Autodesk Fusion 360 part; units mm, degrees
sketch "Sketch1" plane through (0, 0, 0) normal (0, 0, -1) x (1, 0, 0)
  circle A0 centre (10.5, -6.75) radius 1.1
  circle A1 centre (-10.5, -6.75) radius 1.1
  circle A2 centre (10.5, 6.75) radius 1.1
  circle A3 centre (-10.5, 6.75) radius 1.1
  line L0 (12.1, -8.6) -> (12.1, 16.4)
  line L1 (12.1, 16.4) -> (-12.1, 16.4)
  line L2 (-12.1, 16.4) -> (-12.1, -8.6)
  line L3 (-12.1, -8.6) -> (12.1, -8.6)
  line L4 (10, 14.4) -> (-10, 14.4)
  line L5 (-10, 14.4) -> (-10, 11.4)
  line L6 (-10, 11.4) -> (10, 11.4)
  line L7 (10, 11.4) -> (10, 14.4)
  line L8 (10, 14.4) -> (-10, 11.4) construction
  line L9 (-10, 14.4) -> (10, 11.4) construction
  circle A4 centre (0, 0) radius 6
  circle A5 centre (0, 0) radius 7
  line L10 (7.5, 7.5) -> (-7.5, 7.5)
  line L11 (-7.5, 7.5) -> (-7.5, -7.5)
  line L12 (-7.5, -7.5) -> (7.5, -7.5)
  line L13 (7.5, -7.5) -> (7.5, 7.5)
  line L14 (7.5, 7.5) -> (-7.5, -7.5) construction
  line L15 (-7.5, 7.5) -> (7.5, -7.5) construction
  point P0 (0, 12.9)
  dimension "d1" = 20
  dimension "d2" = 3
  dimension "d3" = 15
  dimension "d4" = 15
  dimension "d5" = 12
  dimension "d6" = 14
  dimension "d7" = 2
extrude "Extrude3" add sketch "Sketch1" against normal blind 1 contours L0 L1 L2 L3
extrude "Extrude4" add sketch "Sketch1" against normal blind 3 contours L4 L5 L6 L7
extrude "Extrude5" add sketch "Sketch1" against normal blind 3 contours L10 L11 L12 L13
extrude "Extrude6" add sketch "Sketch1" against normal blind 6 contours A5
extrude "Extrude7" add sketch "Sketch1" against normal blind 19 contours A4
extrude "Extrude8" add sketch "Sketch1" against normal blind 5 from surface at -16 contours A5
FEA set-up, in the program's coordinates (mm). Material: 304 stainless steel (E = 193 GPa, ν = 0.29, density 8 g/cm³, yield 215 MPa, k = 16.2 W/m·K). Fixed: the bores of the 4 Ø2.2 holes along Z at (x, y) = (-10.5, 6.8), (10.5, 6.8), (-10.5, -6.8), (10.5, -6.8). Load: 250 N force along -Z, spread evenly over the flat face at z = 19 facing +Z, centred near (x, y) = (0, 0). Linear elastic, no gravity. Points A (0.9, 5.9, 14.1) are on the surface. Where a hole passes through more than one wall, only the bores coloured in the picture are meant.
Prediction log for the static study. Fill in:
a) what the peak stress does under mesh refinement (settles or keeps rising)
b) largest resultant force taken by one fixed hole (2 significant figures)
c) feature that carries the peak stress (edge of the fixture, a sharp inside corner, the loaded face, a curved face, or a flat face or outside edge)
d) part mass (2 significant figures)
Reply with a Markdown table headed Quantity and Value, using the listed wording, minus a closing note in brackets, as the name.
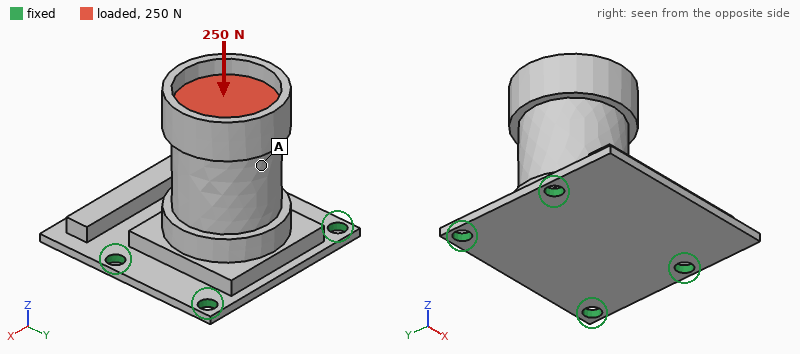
| Quantity | Value |
|---|---|
| what the peak stress does under mesh refinement | keeps rising |
| largest resultant force taken by one fixed hole | 82 N |
| feature that carries the peak stress | edge of the fixture |
| part mass | 26 g |
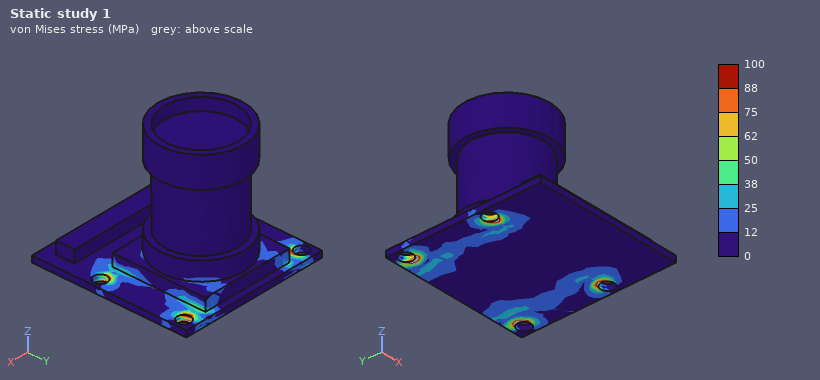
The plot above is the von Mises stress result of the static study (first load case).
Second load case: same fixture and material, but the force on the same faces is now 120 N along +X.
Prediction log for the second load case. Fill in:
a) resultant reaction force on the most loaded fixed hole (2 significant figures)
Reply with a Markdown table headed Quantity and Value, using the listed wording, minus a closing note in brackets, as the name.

| Quantity | Value |
|---|---|
| resultant reaction force on the most loaded fixed hole | 75 N |
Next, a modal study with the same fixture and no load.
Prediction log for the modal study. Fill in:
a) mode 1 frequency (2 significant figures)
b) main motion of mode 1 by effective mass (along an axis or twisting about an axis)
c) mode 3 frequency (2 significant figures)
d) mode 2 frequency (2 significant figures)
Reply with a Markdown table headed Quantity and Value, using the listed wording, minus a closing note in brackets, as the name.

| Quantity | Value |
|---|---|
| mode 1 frequency | 5700 Hz |
| main motion of mode 1 by effective mass | along Y |
| mode 3 frequency | 7800 Hz |
| mode 2 frequency | 7800 Hz |
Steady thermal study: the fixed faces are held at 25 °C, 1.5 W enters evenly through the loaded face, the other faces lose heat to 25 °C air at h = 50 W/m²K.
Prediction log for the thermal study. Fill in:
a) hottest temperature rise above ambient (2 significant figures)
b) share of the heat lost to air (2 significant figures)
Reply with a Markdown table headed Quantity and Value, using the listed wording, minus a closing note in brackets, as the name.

| Quantity | Value |
|---|---|
| hottest temperature rise above ambient | 17 K |
| share of the heat lost to air | 55 % |
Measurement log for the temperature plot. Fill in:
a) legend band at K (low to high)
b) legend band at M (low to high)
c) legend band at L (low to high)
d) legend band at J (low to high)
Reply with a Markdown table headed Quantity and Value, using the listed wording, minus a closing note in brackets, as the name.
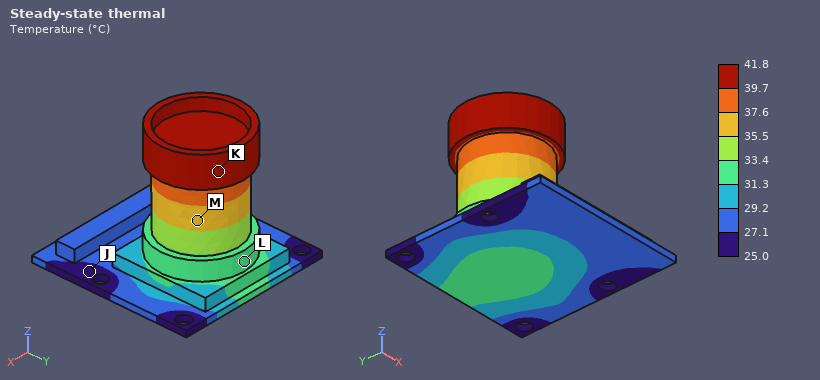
| Quantity | Value |
|---|---|
| legend band at K | 39.7 to 41.8 °C |
| legend band at M | 35.5 to 37.6 °C |
| legend band at L | 31.3 to 33.4 °C |
| legend band at J | 25.0 to 27.1 °C |
